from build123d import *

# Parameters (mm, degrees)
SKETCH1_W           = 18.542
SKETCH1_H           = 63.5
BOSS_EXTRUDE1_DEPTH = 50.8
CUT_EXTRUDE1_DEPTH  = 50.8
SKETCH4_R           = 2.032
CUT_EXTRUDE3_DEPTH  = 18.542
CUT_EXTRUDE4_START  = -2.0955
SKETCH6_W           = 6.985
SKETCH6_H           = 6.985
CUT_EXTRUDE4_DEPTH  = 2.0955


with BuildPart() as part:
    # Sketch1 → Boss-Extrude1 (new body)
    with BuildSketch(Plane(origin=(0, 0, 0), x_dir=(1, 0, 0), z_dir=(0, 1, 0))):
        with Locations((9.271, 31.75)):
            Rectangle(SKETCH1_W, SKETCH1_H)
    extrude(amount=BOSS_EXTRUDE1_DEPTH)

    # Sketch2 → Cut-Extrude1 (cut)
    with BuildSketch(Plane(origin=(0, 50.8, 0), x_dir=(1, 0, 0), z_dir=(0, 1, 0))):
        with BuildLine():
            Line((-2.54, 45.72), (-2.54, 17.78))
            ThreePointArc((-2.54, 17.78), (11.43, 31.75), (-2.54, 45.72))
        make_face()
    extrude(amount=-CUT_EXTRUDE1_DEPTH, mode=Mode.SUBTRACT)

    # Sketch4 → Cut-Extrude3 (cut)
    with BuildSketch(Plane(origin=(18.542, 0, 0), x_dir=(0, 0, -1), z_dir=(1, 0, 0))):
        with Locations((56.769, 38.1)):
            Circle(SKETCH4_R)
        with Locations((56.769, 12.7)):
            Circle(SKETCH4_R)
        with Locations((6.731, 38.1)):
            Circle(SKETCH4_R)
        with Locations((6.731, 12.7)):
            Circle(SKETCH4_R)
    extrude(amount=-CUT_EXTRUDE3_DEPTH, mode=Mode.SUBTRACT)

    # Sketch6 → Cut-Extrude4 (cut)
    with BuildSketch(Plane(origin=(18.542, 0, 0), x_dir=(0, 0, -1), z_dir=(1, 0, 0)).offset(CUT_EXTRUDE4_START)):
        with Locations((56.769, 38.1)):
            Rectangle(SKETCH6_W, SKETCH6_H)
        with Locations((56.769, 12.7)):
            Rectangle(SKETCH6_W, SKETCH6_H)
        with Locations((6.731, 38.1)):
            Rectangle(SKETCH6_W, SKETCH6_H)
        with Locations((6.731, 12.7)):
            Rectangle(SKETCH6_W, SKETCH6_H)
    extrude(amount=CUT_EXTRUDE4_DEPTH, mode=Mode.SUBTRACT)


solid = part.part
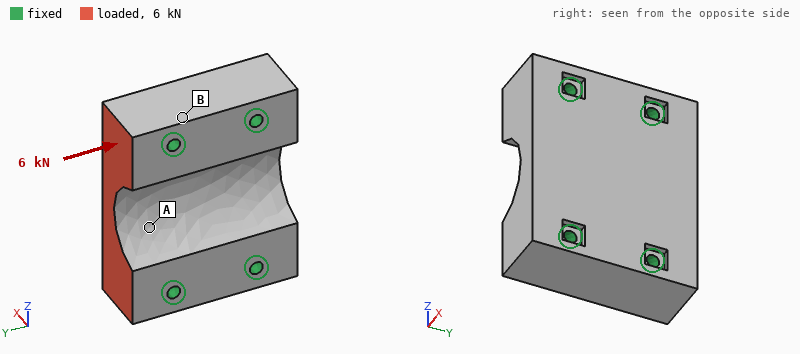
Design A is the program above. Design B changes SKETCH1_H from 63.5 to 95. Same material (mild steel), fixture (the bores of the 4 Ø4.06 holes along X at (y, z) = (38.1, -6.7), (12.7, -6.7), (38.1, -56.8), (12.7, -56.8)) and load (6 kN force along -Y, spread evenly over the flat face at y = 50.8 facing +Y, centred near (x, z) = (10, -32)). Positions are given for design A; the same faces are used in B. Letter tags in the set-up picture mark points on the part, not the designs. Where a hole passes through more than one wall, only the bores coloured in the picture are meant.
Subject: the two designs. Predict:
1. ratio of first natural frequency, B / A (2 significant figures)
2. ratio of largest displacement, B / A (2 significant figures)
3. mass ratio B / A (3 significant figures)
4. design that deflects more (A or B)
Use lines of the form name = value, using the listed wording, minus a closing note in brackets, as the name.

ratio of first natural frequency, B / A = 0.74
ratio of largest displacement, B / A = 0.68
mass ratio B / A = 1.64
design that deflects more = A
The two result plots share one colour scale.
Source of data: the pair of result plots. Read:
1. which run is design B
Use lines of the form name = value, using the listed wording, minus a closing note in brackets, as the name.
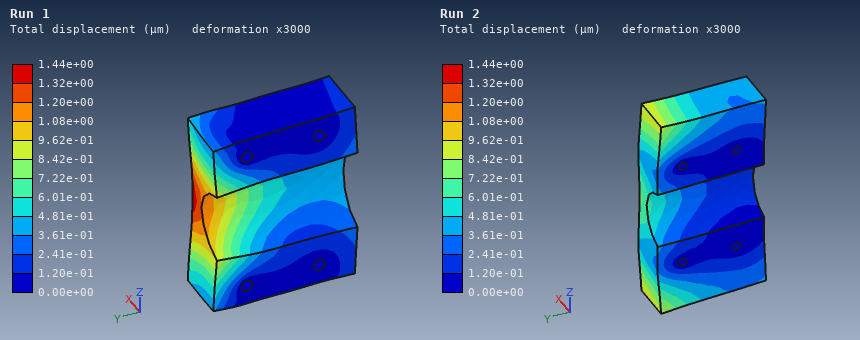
which run is design B = Run 2
